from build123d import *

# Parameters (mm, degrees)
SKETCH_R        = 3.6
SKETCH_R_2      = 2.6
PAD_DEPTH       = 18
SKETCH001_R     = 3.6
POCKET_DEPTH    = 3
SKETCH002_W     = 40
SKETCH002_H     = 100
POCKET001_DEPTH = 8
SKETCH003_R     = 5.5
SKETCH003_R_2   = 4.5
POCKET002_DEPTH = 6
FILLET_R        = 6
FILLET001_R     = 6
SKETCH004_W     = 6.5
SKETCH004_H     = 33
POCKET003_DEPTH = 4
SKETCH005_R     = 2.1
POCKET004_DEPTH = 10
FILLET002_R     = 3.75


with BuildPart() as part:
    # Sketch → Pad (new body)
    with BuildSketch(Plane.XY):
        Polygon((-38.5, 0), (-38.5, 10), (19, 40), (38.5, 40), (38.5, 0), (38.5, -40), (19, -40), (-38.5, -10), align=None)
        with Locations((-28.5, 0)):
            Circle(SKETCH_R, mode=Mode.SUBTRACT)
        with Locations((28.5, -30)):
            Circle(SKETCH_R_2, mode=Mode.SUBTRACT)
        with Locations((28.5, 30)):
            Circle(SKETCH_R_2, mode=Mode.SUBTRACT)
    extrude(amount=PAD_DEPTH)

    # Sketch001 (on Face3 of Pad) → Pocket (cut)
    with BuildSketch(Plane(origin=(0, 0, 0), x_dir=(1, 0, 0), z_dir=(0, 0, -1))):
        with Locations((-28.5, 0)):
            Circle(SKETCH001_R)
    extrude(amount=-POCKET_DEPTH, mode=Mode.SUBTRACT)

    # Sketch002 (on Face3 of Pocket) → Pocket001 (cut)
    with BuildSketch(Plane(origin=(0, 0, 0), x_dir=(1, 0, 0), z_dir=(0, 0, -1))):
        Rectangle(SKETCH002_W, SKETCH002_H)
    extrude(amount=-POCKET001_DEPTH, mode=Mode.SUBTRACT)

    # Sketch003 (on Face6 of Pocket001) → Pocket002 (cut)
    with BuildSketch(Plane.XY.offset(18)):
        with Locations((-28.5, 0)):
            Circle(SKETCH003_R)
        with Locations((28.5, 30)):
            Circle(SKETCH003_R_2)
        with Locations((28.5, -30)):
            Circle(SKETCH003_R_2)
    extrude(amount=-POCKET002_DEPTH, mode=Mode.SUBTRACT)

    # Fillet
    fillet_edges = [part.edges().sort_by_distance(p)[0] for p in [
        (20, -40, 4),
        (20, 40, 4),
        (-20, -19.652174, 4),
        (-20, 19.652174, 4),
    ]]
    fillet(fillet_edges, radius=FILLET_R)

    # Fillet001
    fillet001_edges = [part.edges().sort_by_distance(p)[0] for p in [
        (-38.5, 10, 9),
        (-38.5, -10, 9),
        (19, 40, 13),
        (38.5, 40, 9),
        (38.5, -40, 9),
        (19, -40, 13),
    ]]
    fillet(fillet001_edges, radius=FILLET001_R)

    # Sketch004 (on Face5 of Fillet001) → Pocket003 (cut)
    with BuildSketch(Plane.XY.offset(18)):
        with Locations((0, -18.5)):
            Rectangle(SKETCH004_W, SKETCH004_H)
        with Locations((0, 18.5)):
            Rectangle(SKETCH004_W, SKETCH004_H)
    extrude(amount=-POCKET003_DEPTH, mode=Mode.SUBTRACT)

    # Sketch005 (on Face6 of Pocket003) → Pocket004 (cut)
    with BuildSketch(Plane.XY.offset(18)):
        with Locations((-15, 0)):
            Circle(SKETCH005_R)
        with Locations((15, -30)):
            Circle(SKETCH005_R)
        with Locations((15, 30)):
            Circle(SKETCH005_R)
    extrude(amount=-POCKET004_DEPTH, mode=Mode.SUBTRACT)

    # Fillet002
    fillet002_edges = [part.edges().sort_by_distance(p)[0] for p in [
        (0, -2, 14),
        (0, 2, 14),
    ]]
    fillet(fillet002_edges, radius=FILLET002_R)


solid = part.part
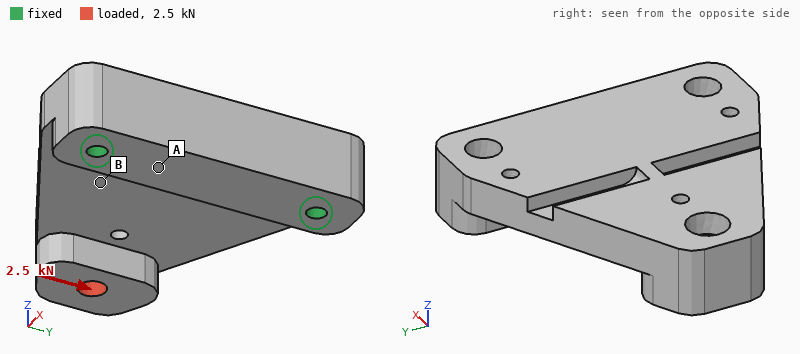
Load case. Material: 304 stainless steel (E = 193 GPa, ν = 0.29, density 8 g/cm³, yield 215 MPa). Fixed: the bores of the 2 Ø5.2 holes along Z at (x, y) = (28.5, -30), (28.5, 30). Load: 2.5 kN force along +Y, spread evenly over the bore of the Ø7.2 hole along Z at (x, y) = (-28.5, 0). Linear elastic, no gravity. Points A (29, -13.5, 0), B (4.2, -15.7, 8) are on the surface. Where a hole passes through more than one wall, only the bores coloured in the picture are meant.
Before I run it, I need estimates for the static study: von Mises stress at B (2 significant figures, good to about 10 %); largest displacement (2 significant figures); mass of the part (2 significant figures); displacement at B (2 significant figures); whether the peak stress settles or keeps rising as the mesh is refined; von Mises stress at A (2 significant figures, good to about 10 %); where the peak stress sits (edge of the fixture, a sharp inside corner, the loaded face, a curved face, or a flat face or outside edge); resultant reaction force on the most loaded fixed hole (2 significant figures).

18 MPa
21 µm
440 g
4.1 µm
keeps rising
6.4 MPa
edge of the fixture
2.6 kN
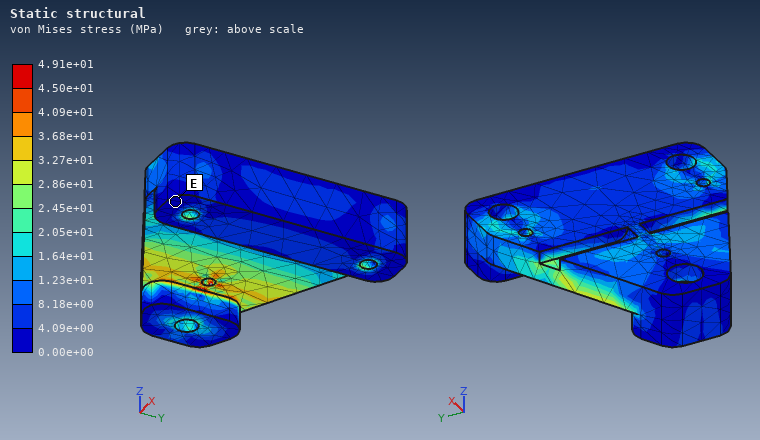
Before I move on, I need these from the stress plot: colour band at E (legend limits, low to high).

0.00e+00 to 4.09e+00 MPa
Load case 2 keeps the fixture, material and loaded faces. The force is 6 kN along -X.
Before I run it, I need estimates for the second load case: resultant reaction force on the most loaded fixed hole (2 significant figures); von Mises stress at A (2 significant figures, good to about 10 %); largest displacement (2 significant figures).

3.1 kN
11 MPa
0.13 mm
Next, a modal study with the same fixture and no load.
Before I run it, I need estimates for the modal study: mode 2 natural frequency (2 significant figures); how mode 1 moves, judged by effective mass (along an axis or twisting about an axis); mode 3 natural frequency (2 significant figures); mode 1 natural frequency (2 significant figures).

6300 Hz
along Z
7400 Hz
1700 Hz
